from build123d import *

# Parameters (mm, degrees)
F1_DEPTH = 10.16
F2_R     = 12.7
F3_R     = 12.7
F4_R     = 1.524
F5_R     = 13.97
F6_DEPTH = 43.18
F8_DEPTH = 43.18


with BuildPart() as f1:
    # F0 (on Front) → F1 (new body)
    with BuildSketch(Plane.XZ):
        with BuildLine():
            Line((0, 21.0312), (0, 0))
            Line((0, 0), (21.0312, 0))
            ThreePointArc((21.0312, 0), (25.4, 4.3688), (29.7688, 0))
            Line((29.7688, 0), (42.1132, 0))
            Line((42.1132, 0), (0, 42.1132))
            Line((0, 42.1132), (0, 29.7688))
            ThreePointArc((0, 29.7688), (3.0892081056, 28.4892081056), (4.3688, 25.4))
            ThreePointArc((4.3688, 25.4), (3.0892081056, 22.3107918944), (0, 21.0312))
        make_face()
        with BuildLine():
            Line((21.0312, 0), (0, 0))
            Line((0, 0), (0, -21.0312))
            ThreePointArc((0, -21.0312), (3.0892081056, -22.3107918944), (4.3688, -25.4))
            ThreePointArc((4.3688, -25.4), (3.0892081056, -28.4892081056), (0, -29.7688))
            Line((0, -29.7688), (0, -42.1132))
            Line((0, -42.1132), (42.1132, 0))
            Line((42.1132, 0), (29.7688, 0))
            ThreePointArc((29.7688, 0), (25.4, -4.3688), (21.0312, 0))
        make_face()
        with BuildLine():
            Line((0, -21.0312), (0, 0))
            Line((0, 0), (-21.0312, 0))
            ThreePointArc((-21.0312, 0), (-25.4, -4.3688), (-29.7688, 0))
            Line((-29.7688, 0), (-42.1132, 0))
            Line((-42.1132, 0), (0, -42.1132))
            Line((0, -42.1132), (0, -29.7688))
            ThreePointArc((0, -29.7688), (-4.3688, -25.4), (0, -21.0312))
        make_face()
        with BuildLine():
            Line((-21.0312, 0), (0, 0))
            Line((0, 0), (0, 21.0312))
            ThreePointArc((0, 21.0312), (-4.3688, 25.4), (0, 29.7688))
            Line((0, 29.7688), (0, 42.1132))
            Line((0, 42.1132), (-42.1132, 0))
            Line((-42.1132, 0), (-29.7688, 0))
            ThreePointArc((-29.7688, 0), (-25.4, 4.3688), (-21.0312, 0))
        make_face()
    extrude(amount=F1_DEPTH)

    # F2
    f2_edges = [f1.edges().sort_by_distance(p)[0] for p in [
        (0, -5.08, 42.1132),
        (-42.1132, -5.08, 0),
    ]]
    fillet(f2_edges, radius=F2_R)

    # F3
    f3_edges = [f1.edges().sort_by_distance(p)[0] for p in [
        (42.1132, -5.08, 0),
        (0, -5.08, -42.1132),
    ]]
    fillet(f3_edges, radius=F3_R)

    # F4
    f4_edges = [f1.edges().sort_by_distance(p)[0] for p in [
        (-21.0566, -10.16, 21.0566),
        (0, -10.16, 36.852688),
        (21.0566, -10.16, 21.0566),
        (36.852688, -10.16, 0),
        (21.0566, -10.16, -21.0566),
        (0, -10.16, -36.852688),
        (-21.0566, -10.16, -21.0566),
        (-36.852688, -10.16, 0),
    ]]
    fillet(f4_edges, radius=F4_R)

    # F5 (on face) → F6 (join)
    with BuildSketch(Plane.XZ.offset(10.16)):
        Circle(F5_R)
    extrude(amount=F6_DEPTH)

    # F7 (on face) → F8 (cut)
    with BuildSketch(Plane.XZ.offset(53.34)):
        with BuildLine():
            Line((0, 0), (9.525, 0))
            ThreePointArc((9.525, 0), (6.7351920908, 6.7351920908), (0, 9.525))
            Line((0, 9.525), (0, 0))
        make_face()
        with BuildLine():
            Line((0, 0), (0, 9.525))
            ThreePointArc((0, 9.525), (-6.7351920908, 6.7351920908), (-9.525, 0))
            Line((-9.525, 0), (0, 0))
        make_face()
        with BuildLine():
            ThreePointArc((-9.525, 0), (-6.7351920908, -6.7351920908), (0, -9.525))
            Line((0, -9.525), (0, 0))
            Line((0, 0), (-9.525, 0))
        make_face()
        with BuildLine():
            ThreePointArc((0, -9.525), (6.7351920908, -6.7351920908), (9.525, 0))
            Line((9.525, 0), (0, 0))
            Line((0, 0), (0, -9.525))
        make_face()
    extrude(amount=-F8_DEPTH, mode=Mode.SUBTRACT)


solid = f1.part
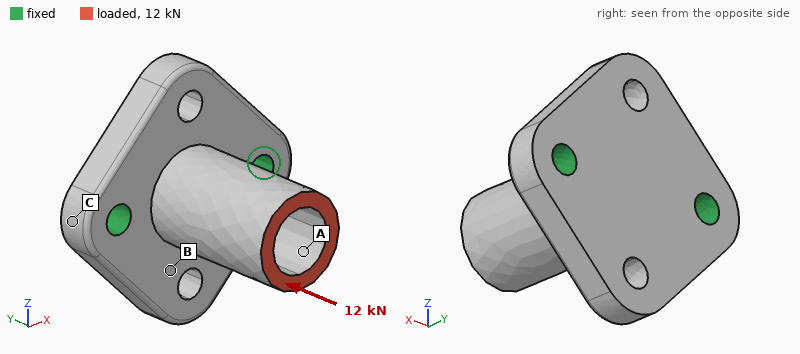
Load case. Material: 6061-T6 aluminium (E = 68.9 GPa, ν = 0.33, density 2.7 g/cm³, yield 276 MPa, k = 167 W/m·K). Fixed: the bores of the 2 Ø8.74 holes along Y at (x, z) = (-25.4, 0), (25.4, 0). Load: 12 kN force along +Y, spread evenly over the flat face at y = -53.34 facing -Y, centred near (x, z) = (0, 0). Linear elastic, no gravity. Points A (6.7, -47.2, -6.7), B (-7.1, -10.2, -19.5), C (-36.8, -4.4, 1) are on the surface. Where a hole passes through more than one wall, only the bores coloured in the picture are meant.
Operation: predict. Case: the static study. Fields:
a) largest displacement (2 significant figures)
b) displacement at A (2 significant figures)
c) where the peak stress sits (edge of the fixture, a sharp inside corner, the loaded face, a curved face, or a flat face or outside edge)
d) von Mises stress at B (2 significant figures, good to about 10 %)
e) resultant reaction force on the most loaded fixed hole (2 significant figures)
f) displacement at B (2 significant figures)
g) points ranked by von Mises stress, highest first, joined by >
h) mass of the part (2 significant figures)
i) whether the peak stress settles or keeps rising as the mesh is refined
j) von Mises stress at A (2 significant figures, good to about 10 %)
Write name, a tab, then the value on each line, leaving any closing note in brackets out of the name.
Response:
largest displacement	49 µm
displacement at A	45 µm
where the peak stress sits	edge of the fixture
von Mises stress at B	22 MPa
resultant reaction force on the most loaded fixed hole	6.1 kN
displacement at B	28 µm
points ranked by von Mises stress, highest first, joined by >	A > B > C
mass of the part	120 g
whether the peak stress settles or keeps rising as the mesh is refined	keeps rising
von Mises stress at A	37 MPa
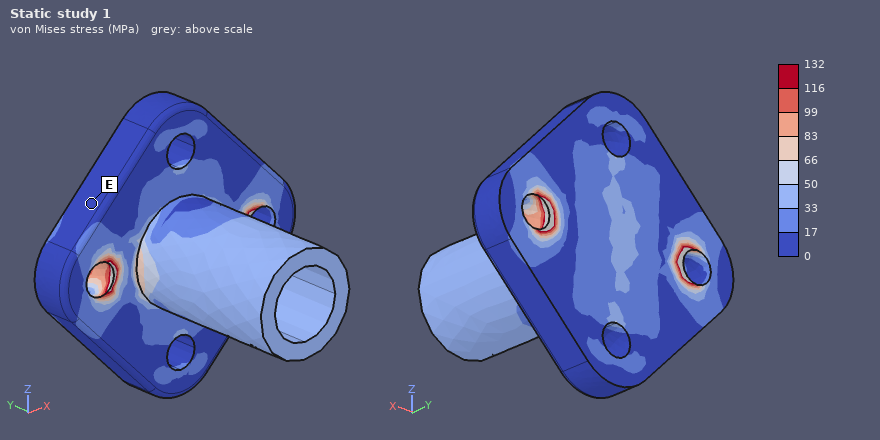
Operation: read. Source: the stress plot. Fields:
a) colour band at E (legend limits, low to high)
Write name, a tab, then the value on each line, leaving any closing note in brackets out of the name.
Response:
colour band at E	0 to 17 MPa
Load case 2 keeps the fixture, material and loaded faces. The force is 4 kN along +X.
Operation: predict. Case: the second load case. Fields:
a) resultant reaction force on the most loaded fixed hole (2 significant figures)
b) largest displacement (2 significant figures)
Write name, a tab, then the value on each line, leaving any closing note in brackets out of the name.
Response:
resultant reaction force on the most loaded fixed hole	5.3 kN
largest displacement	0.17 mm
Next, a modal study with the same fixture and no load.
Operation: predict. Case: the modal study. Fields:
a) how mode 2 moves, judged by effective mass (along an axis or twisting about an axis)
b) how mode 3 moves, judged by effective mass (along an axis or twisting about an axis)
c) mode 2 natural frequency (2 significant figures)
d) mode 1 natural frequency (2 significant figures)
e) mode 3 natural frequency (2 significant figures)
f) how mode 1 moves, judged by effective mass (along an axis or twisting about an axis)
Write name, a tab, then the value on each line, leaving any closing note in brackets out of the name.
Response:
how mode 2 moves, judged by effective mass	along X
how mode 3 moves, judged by effective mass	along Y
mode 2 natural frequency	7200 Hz
mode 1 natural frequency	4200 Hz
mode 3 natural frequency	9000 Hz
how mode 1 moves, judged by effective mass	along Z
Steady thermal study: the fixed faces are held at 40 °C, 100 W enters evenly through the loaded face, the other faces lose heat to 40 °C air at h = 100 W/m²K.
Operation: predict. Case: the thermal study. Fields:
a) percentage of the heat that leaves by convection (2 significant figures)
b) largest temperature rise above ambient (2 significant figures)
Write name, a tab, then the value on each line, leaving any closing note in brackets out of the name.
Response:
percentage of the heat that leaves by convection	32 %
largest temperature rise above ambient	77 K
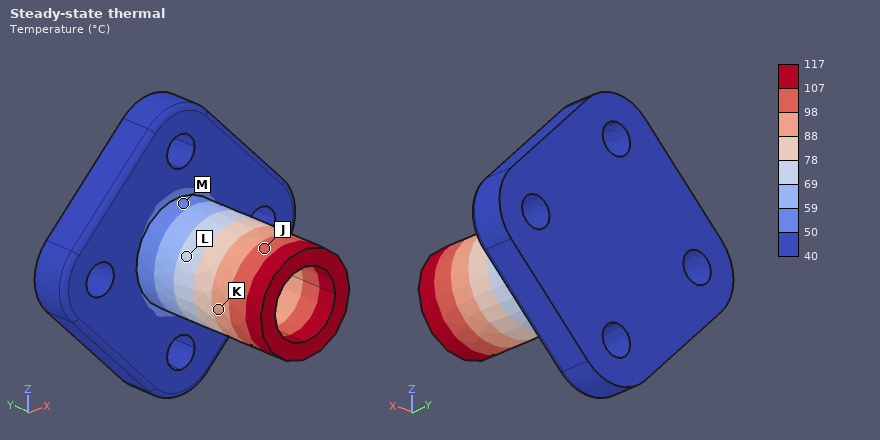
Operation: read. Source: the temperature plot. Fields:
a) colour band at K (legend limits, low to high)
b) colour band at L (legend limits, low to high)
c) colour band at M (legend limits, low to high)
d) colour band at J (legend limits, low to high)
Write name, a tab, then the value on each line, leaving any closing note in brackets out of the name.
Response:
colour band at K	88 to 98 °C
colour band at L	69 to 78 °C
colour band at M	50 to 59 °C
colour band at J	98 to 107 °C
